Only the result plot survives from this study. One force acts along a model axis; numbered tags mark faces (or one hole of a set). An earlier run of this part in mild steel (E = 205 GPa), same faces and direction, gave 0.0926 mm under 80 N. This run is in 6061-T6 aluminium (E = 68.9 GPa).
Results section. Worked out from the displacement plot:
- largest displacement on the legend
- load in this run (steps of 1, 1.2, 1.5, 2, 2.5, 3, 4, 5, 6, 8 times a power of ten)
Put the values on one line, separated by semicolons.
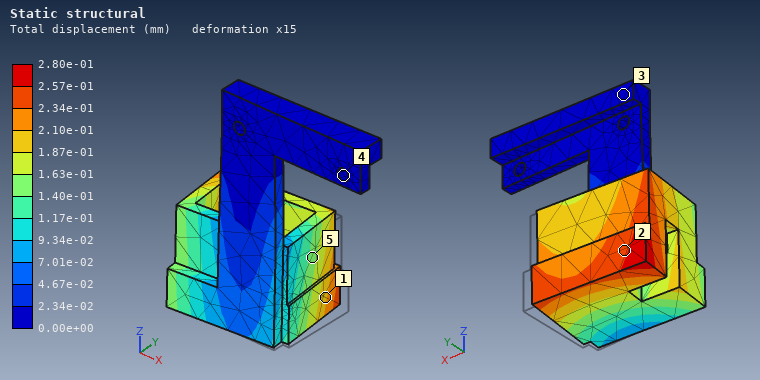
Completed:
2.80e-01 mm; 80 N
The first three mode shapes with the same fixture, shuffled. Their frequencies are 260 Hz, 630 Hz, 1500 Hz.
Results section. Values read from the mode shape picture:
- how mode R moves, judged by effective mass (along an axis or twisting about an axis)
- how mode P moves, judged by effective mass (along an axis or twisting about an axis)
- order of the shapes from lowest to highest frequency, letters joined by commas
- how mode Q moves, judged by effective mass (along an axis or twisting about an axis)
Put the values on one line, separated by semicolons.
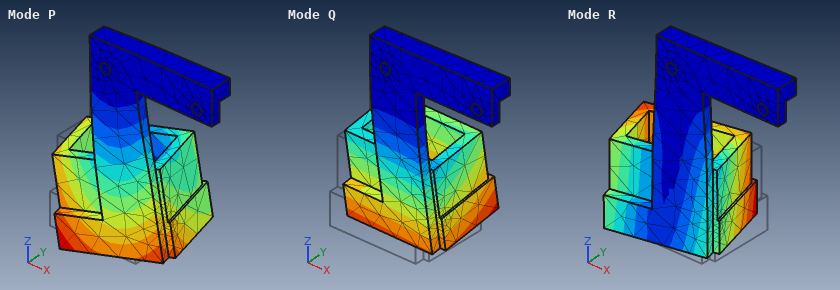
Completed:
along X; along X; Q, R, P; along Y
